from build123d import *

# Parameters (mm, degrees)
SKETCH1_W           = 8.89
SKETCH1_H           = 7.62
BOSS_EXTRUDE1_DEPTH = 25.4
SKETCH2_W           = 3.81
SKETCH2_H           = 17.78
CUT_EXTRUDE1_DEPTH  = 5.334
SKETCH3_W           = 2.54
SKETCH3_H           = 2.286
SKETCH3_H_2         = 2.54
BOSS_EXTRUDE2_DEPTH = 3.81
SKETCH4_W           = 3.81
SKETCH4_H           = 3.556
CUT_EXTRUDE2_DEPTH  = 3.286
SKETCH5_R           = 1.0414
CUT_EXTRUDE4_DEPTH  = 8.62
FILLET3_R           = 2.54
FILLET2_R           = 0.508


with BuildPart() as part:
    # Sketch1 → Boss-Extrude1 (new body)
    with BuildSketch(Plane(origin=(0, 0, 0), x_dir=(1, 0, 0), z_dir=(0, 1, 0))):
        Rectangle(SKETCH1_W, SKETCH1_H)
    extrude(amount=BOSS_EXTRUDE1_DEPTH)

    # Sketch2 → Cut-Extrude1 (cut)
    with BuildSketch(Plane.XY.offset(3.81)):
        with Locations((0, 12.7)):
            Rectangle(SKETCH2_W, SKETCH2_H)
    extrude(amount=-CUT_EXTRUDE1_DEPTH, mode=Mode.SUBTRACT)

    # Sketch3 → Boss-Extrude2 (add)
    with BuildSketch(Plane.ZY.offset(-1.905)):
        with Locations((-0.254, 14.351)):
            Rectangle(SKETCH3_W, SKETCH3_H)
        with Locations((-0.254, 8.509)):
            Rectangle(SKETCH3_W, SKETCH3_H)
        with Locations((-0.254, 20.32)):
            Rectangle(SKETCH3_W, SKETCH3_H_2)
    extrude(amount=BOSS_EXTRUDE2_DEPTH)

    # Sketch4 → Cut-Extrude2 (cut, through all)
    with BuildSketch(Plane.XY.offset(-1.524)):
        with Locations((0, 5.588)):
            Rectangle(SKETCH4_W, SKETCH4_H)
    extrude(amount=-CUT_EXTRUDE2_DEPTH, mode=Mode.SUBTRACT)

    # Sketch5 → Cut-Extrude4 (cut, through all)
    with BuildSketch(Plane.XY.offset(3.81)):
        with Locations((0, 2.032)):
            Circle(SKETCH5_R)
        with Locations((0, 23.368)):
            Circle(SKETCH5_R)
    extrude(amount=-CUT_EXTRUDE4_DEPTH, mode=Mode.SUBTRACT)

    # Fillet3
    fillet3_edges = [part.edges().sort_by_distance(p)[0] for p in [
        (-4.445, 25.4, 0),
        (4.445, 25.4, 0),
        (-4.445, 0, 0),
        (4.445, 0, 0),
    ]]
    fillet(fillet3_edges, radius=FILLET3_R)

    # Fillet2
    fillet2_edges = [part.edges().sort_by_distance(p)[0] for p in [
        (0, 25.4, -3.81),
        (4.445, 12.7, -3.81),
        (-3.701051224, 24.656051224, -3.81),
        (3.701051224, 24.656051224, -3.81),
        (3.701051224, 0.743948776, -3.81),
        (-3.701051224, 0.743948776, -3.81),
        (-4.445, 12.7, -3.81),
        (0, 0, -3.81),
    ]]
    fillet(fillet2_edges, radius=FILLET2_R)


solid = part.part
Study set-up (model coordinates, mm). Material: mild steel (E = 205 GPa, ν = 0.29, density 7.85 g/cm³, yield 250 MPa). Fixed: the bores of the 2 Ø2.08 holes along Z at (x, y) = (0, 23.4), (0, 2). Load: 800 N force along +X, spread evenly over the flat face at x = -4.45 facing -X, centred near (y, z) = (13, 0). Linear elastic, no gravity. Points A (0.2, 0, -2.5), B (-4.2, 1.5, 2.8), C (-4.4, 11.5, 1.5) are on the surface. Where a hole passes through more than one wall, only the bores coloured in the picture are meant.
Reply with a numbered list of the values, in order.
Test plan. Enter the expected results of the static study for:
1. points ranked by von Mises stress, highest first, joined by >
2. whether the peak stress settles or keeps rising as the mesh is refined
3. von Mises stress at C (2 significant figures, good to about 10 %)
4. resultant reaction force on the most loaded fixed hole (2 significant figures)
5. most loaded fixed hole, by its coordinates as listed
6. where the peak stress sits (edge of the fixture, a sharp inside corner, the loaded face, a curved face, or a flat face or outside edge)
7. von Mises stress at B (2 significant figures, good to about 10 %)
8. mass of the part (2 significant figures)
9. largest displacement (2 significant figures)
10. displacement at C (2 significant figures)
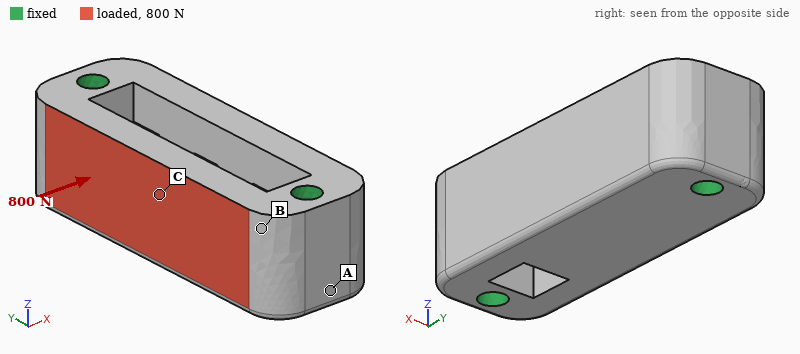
1. C > B > A
2. keeps rising
3. 32 MPa
4. 430 N
5. (0, 23.4)
6. edge of the fixture
7. 14 MPa
8. 10 g
9. 4.2 µm
10. 3.3 µm
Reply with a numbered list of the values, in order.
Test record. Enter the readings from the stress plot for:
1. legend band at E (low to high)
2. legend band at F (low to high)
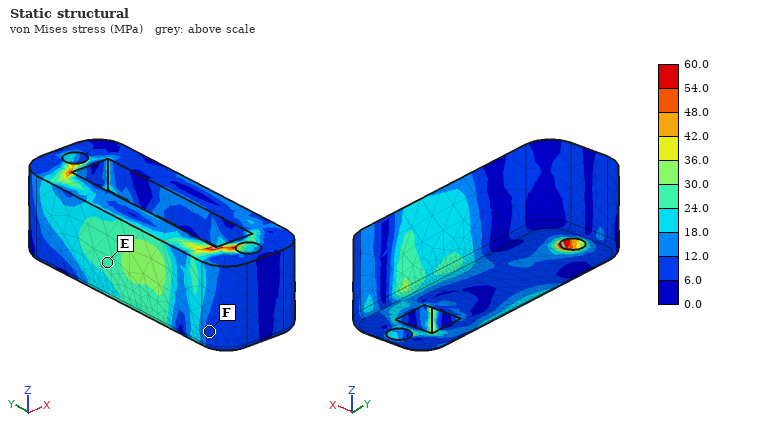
1. 24.0 to 30.0 MPa
2. 6.0 to 12.0 MPa
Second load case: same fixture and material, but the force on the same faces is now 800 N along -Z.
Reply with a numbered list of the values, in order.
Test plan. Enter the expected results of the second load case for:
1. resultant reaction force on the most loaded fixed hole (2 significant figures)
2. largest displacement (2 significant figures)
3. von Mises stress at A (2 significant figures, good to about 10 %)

1. 420 N
2. 4.5 µm
3. 14 MPa
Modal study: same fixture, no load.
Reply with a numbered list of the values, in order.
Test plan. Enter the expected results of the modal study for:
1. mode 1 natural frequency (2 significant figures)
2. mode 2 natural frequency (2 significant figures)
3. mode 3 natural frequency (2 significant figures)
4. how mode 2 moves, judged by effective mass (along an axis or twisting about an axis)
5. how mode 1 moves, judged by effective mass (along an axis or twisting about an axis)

1. 36 kHz
2. 45 kHz
3. 53 kHz
4. along Z
5. along X
